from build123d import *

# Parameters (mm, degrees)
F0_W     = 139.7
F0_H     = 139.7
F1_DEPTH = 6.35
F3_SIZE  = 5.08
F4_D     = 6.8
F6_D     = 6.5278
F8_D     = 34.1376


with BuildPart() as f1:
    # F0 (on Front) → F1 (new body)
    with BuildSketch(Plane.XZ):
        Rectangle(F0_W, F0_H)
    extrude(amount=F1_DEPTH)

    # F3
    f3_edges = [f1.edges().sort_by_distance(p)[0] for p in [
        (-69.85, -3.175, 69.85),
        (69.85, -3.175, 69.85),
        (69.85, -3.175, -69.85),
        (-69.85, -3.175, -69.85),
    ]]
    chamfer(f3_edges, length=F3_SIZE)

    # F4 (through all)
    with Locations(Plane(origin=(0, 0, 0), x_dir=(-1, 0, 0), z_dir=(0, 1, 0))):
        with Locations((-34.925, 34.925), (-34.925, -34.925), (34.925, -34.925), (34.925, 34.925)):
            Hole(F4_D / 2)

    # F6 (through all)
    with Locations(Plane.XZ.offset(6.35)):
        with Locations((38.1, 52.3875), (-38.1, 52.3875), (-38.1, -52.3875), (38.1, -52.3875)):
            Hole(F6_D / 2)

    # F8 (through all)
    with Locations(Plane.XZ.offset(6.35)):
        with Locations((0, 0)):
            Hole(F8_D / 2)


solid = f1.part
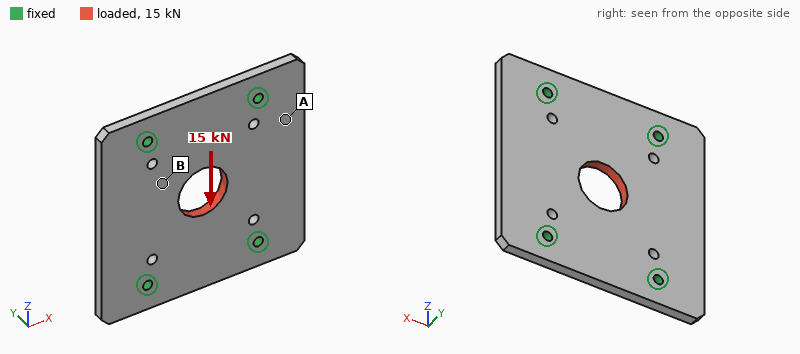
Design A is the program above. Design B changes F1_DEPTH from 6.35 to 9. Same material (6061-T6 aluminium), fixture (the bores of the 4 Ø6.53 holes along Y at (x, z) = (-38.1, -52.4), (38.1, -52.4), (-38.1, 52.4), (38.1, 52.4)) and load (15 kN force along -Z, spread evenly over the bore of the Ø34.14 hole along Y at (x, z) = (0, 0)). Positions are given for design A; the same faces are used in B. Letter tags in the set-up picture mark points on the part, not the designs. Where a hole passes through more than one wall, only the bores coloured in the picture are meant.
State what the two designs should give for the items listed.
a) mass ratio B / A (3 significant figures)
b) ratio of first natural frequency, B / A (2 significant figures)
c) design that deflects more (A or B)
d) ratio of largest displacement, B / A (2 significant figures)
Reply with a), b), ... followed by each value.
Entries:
a) 1.42
b) 1.3
c) A
d) 0.70
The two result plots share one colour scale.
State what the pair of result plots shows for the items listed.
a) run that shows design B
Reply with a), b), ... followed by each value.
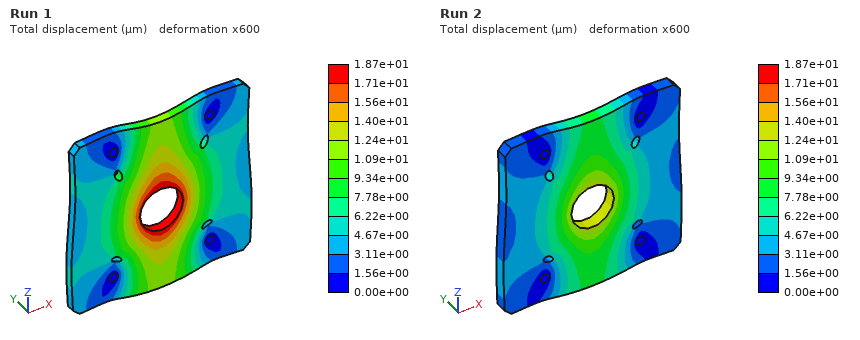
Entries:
a) Run 2
